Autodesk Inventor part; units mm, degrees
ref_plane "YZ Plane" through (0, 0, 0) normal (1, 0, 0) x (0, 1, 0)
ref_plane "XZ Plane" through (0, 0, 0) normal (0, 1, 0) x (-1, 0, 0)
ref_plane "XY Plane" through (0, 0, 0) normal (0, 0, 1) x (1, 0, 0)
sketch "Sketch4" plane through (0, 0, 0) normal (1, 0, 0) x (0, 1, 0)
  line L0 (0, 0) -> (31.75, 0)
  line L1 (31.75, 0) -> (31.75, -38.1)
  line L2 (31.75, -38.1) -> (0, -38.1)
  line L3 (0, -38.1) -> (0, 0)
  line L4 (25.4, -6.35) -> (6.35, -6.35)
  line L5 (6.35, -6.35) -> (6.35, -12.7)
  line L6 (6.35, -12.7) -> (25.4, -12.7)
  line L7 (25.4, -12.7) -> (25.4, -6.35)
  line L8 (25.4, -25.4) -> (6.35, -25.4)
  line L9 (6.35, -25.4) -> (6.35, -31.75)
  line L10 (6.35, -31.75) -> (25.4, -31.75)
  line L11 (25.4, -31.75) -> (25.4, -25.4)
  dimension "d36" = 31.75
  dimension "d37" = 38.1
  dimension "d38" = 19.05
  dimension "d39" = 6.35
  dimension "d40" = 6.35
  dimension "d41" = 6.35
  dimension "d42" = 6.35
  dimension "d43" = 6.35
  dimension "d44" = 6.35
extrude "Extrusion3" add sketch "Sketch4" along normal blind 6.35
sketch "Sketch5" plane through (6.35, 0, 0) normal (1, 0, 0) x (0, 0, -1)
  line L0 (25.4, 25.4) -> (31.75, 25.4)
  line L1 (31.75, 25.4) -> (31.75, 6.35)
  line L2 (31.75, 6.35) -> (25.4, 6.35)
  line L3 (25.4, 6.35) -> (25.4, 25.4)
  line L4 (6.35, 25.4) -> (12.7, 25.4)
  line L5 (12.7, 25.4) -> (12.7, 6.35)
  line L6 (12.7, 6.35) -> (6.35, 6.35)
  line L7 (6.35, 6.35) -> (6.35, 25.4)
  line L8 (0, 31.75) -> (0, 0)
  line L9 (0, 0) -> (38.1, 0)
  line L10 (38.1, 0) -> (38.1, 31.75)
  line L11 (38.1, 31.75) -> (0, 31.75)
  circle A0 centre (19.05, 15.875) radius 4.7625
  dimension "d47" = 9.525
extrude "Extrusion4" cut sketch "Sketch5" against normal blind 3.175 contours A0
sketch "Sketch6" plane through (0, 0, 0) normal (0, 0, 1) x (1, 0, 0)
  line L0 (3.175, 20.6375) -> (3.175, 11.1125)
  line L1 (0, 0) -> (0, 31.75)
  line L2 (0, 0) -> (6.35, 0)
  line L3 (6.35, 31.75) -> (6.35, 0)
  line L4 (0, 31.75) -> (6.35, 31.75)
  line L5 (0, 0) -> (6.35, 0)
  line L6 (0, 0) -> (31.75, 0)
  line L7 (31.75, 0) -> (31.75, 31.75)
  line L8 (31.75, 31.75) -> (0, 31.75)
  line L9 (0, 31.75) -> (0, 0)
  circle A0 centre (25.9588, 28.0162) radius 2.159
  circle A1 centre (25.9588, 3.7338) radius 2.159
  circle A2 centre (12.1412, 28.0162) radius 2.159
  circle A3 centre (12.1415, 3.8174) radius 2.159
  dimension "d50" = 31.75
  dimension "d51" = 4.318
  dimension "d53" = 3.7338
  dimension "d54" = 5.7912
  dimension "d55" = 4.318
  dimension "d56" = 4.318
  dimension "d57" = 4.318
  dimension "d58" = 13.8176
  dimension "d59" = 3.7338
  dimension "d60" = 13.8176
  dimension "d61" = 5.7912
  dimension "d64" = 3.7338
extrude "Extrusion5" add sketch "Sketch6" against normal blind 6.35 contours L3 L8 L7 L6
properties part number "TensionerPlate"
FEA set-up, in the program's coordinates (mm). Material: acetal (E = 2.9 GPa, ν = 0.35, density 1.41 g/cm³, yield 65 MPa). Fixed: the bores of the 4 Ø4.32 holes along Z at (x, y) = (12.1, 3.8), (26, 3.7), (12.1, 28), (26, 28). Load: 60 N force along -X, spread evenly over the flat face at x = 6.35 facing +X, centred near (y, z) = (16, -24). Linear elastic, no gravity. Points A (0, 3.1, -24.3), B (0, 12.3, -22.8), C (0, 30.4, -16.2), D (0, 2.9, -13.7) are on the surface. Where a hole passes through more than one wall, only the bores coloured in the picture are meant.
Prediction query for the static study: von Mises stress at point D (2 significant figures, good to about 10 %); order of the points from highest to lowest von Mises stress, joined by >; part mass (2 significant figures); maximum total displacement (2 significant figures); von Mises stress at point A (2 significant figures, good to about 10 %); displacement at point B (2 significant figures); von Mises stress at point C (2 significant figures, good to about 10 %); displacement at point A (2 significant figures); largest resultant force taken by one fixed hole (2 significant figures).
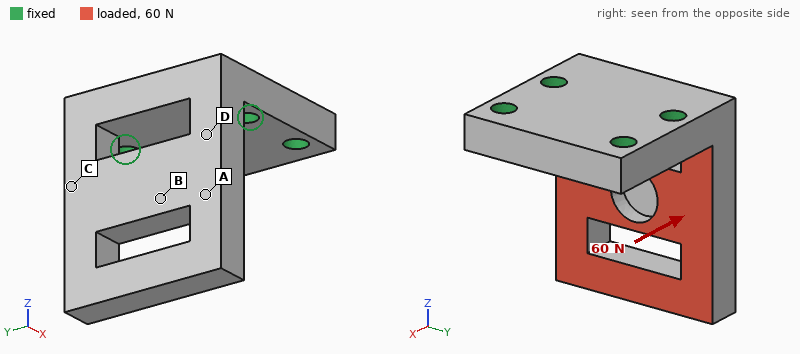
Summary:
6.6 MPa
D > C > A > B
15 g
0.64 mm
2.3 MPa
0.31 mm
5.0 MPa
0.34 mm
30 N
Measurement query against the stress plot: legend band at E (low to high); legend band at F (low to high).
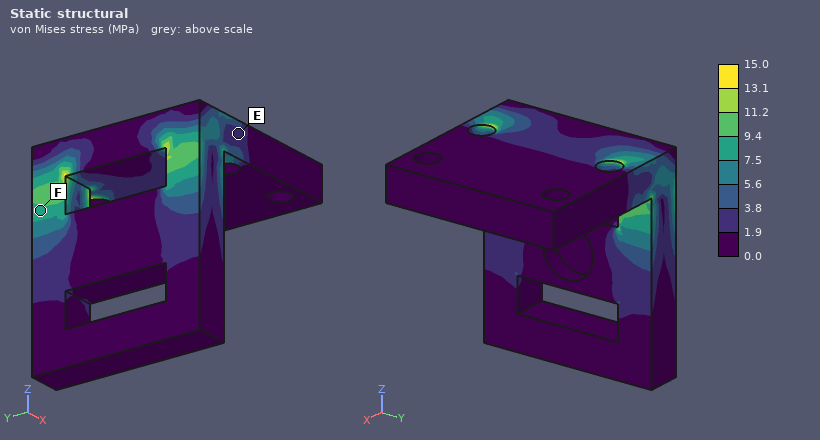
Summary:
1.9 to 3.8 MPa
7.5 to 9.4 MPa
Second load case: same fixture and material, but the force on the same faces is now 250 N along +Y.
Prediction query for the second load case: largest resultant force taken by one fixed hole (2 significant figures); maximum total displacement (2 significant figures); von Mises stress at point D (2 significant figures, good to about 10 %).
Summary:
230 N
0.52 mm
3.8 MPa
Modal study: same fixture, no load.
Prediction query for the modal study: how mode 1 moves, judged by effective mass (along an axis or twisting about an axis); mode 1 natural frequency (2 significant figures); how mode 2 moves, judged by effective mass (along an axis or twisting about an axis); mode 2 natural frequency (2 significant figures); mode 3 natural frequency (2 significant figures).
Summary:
along X
740 Hz
along Y
1800 Hz
2300 Hz
